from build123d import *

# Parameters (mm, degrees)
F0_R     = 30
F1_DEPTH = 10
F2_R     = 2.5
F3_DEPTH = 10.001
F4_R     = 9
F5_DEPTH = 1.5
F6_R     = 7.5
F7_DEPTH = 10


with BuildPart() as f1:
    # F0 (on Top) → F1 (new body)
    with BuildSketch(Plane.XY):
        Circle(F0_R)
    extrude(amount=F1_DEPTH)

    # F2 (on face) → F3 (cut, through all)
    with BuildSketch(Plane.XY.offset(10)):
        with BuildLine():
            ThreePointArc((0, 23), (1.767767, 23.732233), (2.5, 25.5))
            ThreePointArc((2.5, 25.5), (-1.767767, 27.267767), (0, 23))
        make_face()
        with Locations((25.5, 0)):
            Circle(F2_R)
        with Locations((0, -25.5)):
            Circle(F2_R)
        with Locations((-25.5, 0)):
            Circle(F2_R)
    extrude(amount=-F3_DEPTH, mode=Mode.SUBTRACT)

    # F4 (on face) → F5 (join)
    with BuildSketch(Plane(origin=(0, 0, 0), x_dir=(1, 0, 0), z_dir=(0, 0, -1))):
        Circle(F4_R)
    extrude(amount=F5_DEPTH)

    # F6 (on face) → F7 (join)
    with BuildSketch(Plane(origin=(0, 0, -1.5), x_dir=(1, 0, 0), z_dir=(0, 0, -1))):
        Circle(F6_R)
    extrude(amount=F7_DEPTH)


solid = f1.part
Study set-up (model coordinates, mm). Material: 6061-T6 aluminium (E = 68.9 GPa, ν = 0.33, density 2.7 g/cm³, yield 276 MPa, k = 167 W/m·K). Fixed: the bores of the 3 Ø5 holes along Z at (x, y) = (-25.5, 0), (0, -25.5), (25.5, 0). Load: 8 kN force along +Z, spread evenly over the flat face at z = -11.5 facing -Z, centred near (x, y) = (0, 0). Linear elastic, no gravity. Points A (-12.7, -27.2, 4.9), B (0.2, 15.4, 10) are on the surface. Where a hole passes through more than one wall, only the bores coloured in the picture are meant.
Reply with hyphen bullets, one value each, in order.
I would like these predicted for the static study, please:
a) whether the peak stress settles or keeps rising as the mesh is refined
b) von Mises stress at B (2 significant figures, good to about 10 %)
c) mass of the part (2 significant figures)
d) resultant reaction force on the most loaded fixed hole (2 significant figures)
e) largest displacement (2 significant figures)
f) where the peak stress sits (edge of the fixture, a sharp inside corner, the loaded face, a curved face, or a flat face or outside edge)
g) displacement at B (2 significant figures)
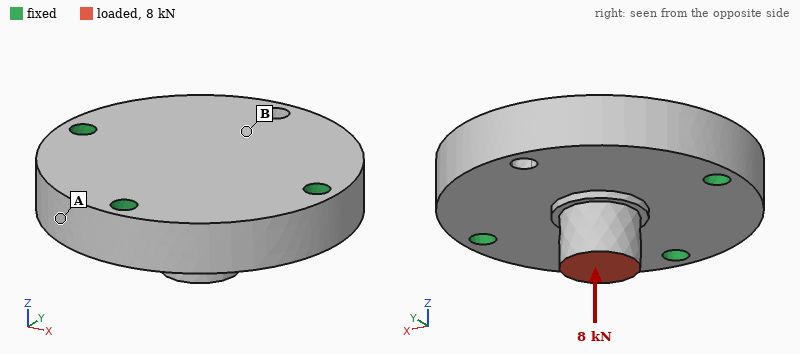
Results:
- keeps rising
- 39 MPa
- 80 g
- 3.2 kN
- 55 µm
- edge of the fixture
- 41 µm
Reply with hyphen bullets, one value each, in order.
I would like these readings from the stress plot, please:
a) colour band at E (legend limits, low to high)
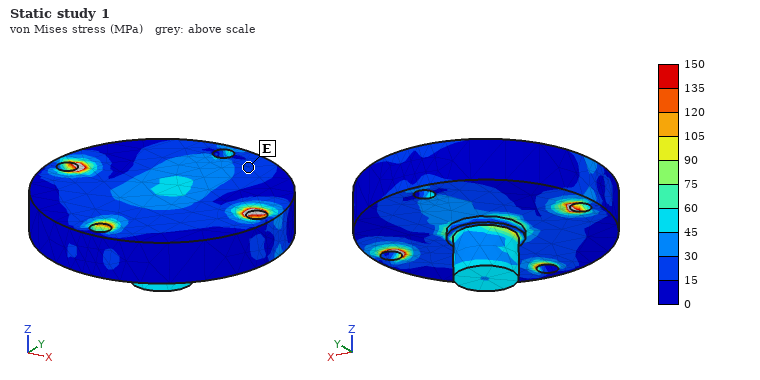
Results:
- 15 to 30 MPa
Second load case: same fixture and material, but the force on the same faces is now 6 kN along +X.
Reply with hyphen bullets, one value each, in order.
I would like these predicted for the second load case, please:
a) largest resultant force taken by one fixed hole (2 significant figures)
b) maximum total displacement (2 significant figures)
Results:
- 3.4 kN
- 70 µm
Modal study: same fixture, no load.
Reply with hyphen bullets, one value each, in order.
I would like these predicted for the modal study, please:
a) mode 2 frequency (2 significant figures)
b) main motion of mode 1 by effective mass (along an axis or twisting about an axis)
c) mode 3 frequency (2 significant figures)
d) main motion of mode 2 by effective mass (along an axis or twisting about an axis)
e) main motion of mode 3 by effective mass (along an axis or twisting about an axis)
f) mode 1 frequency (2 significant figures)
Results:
- 19 kHz
- along Z
- 20 kHz
- twisting about Y
- along Z
- 8000 Hz
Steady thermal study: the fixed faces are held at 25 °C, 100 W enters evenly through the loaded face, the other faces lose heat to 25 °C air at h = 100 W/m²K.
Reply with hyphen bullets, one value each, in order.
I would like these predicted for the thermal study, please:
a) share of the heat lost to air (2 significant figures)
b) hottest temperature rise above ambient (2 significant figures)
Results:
- 8.0 %
- 61 K
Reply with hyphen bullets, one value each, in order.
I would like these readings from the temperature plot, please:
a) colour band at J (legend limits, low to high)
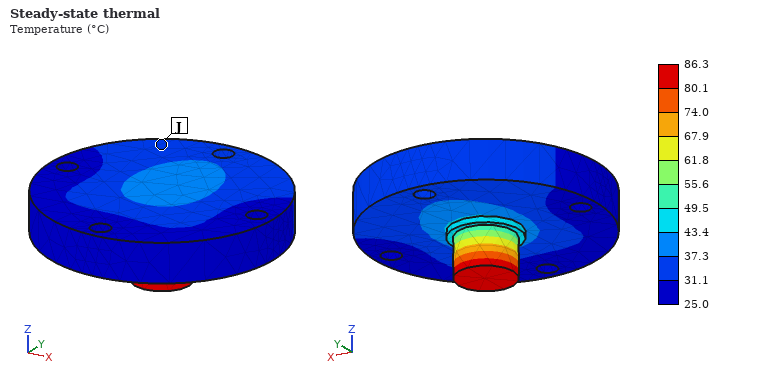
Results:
- 31.1 to 37.3 °C
